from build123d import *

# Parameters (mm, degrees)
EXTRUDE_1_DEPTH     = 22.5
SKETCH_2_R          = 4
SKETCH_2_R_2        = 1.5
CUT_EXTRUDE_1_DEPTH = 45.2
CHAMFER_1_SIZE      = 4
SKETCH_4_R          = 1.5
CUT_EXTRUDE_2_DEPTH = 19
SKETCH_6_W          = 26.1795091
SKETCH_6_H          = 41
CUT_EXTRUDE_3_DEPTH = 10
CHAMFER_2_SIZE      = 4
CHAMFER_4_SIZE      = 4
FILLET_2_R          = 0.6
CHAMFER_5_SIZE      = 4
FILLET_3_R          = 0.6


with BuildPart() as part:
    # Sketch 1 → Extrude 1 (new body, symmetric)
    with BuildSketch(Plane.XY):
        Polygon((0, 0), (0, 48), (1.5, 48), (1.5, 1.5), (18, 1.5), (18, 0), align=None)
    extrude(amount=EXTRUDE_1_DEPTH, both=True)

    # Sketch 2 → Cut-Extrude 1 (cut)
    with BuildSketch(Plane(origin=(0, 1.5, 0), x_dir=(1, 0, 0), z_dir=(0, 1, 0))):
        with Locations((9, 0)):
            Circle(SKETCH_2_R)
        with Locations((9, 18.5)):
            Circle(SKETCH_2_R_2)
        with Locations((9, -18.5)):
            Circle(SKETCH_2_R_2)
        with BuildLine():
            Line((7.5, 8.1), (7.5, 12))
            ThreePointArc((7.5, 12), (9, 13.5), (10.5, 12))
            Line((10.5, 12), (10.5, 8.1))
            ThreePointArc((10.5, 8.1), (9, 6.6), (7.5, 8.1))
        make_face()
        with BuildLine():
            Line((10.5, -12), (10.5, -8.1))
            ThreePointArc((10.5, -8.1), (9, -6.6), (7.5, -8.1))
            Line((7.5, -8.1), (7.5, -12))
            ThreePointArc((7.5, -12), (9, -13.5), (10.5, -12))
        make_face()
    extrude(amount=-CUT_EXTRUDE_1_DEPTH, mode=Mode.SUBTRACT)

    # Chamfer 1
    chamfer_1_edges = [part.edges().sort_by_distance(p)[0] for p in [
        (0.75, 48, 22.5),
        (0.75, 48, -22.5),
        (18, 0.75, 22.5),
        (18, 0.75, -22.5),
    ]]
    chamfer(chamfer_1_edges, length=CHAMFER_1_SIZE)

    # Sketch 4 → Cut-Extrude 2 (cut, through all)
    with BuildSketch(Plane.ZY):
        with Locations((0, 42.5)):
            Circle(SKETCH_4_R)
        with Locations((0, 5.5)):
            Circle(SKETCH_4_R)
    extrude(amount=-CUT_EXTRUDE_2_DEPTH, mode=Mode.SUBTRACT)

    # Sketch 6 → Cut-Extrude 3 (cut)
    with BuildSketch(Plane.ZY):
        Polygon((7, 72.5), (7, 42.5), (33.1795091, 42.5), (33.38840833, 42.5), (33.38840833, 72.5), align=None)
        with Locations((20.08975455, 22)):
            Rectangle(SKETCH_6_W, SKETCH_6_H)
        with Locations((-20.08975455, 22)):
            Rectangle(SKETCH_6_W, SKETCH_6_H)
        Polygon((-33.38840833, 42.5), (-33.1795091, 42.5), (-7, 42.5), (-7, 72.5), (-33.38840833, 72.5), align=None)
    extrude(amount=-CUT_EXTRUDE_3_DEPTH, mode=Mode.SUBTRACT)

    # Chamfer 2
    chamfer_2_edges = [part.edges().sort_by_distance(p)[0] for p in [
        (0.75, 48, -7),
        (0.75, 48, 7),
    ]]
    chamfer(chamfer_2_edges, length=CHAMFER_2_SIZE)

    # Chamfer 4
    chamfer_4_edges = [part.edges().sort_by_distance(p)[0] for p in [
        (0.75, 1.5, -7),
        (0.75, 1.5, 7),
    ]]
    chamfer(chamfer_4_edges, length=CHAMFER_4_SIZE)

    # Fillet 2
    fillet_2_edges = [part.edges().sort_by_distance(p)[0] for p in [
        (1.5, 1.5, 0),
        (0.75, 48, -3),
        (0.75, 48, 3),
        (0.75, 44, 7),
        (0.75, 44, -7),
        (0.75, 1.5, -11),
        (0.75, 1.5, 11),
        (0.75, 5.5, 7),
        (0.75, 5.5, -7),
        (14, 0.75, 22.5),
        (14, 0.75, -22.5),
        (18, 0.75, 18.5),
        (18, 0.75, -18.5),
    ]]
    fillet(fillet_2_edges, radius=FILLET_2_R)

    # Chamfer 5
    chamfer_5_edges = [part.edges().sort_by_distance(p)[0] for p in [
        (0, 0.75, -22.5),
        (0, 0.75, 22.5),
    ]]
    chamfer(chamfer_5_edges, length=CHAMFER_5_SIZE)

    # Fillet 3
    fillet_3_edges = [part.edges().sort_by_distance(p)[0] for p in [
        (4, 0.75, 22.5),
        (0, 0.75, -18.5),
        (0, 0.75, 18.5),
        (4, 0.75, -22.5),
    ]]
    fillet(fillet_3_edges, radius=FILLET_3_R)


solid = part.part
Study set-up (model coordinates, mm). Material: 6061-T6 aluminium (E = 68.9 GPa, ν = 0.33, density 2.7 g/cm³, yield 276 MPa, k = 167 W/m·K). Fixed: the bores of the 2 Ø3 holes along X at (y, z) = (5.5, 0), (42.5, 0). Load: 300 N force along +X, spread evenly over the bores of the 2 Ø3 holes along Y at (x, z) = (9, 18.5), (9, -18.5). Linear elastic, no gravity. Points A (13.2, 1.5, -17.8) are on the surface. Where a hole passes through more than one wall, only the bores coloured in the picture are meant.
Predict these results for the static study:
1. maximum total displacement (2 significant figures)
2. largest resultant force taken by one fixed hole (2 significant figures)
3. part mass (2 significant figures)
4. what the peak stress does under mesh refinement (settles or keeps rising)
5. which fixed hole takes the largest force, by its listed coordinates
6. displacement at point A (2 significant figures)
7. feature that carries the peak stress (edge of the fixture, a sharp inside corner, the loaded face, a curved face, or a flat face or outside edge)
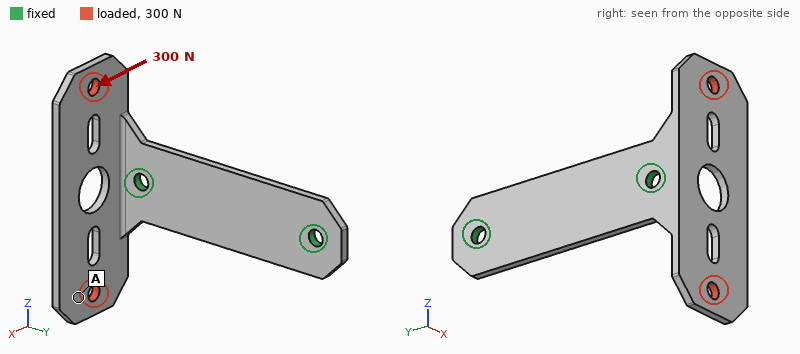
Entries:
0.16 mm
300 N
5.3 g
keeps rising
(5.5, 0)
0.12 mm
edge of the fixture
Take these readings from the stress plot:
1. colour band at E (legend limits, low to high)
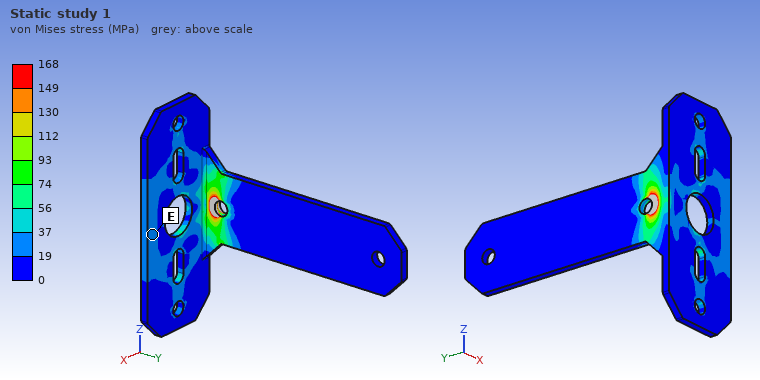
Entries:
19 to 37 MPa
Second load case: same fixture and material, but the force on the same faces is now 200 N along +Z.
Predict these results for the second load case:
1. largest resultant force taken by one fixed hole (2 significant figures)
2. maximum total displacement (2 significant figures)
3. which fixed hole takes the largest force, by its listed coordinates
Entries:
220 N
0.30 mm
(5.5, 0)
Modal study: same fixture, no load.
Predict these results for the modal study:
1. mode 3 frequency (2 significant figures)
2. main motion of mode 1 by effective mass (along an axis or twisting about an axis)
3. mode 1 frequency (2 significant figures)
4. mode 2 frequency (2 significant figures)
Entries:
2900 Hz
along Y
2000 Hz
2100 Hz
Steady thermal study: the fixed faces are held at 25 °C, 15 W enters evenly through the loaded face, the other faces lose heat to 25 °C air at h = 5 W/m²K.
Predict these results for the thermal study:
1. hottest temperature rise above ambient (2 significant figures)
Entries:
66 K
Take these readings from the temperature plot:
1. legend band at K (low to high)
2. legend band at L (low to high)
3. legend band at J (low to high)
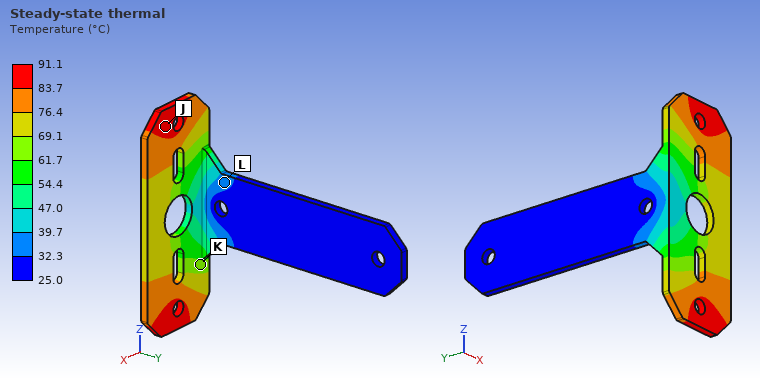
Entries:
61.7 to 69.1 °C
32.3 to 39.7 °C
83.7 to 91.1 °C
